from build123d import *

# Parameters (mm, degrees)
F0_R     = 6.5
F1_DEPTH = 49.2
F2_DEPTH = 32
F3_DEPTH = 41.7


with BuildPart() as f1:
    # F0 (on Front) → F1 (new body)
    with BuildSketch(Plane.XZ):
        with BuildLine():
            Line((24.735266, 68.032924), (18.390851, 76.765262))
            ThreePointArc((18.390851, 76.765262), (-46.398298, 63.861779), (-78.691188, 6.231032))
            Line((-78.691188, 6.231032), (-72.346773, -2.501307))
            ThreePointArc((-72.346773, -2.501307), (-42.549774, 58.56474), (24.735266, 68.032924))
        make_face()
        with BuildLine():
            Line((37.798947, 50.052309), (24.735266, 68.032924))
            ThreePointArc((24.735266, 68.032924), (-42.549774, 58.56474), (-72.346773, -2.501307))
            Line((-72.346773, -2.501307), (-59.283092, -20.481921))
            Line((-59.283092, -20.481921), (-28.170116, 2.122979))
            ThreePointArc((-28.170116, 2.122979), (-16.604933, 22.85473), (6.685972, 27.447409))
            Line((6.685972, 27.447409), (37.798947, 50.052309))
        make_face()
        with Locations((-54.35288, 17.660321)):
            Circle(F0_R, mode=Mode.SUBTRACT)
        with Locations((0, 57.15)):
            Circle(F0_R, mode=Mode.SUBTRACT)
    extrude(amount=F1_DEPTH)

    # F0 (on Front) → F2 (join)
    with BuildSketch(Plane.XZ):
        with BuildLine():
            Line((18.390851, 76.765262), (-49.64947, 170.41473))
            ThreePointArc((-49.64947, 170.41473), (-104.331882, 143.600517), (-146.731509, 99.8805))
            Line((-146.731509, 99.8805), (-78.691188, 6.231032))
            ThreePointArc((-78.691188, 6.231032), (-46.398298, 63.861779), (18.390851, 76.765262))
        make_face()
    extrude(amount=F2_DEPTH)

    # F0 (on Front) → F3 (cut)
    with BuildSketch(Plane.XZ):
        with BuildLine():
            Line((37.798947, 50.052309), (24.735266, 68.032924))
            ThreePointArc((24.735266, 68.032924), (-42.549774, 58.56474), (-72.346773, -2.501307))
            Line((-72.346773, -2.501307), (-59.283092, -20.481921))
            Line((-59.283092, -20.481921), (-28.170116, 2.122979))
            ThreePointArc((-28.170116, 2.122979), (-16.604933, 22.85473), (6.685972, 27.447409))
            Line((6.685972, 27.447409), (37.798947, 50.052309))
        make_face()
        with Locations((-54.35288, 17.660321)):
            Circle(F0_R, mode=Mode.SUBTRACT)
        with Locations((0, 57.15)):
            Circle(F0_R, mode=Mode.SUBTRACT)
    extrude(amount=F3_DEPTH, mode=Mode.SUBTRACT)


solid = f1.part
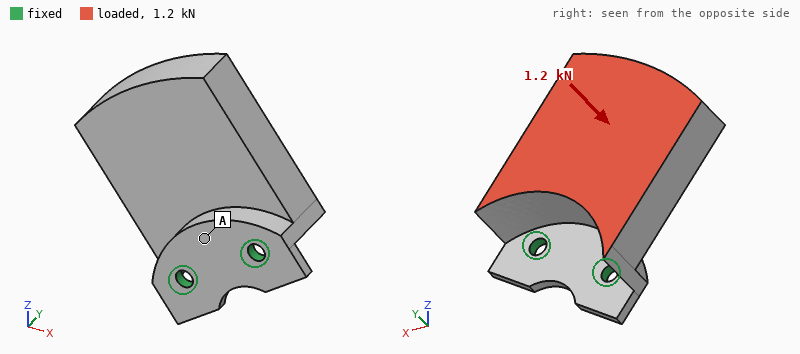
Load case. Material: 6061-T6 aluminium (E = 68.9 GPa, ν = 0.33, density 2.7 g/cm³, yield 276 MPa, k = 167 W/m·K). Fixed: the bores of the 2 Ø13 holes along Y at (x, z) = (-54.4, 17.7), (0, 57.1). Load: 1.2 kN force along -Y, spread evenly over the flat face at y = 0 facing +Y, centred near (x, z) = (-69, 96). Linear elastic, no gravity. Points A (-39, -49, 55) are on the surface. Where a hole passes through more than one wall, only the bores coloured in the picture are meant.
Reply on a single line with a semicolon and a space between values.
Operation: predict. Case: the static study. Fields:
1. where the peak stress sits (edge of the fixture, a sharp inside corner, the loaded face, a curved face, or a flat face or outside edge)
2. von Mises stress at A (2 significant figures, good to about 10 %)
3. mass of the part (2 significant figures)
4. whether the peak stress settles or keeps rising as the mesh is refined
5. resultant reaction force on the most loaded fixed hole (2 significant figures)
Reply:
edge of the fixture; 13 MPa; 1.3 kg; keeps rising; 760 N
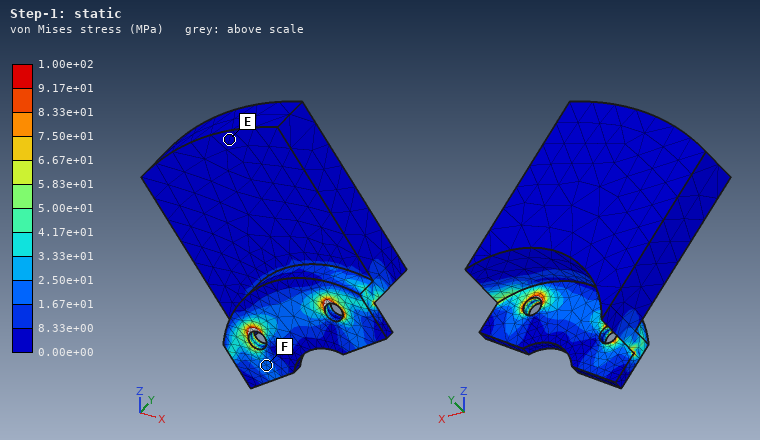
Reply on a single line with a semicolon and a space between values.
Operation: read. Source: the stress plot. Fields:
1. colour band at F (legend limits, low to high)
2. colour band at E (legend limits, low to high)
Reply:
1.67e+01 to 2.50e+01 MPa; 0.00e+00 to 8.33e+00 MPa
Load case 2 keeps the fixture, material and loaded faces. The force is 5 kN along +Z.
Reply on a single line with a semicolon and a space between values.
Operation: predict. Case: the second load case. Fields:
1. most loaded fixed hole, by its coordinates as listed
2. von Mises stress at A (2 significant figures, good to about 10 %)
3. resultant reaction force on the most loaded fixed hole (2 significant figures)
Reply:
(-54.4, 17.7); 36 MPa; 5.1 kN
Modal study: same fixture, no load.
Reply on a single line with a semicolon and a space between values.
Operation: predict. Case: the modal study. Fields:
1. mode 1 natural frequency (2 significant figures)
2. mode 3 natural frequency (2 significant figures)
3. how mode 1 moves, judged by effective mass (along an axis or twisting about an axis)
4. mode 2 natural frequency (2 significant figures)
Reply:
270 Hz; 1700 Hz; along Y; 1300 Hz
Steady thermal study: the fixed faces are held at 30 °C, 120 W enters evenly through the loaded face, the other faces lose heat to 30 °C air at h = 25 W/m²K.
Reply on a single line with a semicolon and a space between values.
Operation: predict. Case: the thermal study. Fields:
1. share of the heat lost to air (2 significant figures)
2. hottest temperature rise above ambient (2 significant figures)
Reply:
20 %; 33 K
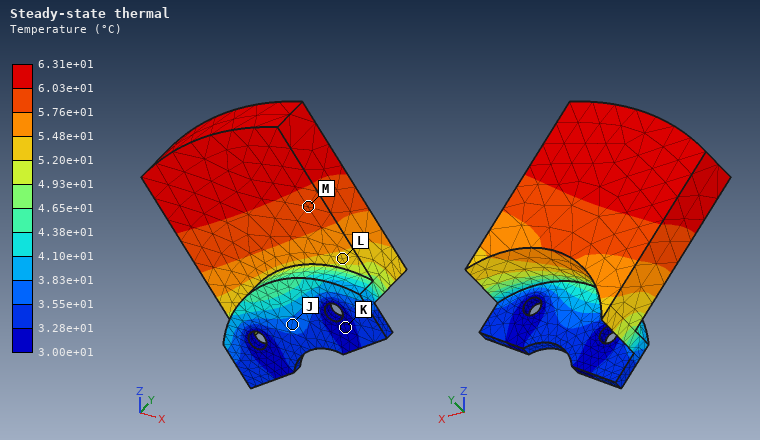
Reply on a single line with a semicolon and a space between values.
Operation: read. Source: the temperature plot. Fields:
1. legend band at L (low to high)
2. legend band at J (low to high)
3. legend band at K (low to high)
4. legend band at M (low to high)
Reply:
5.20e+01 to 5.48e+01 °C; 3.55e+01 to 3.83e+01 °C; 3.00e+01 to 3.28e+01 °C; 5.76e+01 to 6.03e+01 °C
